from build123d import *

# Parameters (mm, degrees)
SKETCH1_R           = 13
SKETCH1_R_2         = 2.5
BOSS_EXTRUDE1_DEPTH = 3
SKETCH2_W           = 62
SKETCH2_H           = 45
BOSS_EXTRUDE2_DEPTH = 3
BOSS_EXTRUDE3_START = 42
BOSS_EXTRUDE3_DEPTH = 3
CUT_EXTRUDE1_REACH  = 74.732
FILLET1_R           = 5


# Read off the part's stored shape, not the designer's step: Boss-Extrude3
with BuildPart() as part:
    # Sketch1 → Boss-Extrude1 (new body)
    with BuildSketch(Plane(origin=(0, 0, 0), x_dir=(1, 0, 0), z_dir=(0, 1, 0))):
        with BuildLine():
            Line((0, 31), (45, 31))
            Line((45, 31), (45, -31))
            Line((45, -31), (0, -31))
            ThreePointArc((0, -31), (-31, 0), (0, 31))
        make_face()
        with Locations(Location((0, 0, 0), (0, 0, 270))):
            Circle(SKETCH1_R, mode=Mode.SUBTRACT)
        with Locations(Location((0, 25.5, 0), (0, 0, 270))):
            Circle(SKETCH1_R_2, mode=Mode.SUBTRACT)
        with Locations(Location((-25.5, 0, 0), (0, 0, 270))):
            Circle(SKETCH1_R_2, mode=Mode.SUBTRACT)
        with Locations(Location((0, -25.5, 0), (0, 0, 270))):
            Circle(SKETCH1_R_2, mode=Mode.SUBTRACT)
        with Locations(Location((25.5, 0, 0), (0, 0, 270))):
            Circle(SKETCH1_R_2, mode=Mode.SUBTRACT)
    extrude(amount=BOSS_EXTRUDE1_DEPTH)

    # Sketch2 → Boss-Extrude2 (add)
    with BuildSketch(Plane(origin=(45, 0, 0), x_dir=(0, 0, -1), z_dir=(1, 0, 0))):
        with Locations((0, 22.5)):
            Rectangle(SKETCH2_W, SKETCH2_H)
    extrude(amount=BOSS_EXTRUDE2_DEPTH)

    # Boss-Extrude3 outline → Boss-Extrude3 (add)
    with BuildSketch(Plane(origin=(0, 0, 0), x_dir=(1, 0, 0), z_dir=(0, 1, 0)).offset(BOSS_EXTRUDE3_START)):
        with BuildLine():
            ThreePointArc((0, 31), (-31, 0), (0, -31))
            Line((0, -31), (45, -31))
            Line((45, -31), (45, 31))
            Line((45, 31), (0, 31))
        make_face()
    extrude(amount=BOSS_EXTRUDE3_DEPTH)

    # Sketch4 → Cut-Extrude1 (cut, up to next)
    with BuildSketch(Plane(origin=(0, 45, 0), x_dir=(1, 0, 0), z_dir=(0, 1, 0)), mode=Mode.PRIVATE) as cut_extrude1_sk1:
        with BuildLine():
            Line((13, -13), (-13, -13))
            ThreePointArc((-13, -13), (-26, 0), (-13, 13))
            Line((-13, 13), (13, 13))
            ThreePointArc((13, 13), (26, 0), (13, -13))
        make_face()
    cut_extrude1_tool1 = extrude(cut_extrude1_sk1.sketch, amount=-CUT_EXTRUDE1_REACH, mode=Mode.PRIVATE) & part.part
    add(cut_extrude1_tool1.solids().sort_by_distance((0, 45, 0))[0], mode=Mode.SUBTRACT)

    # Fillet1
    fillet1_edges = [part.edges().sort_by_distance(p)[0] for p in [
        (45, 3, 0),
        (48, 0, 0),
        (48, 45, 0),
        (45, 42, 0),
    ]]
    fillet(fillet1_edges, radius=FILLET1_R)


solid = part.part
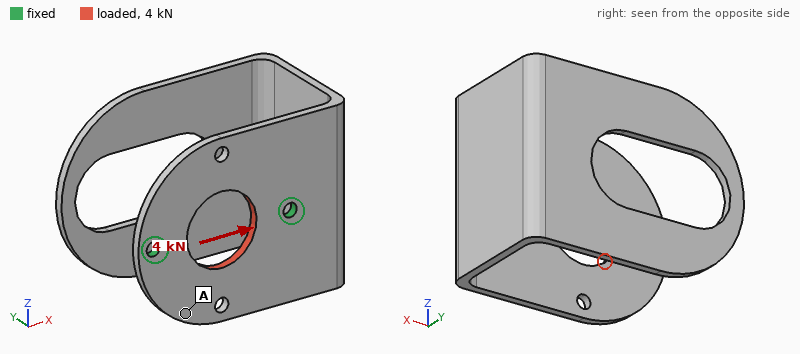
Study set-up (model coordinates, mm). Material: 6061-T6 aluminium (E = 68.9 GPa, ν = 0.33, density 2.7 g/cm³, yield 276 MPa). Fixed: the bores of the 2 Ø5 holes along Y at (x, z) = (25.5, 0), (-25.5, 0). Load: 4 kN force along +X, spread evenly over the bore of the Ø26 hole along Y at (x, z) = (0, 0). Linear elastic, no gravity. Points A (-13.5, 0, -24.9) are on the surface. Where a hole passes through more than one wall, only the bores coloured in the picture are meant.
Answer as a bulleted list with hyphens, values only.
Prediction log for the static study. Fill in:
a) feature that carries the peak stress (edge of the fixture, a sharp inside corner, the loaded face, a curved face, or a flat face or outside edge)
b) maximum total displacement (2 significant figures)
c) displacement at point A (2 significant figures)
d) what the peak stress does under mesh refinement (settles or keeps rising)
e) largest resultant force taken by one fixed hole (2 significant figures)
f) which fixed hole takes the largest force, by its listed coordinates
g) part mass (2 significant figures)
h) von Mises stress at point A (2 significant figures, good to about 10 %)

- edge of the fixture
- 13 µm
- 9.6 µm
- keeps rising
- 2.2 kN
- (25.5, 0)
- 78 g
- 6.2 MPa
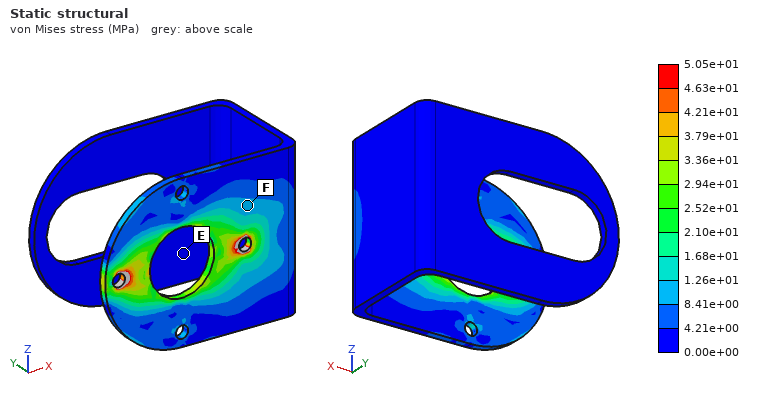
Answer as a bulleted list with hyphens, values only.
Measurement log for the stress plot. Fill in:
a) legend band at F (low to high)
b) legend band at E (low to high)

- 8.41e+00 to 1.26e+01 MPa
- 0.00e+00 to 4.21e+00 MPa
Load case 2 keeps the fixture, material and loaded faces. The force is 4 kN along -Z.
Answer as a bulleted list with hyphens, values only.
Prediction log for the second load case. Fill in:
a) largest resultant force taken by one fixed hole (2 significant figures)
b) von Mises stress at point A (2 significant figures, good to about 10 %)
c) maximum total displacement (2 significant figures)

- 2.0 kN
- 18 MPa
- 16 µm
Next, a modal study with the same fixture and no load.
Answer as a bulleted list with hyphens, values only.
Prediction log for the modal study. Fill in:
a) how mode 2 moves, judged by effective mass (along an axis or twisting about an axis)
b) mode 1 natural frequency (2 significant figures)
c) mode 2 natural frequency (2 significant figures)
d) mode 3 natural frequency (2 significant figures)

- along Z
- 260 Hz
- 380 Hz
- 630 Hz
